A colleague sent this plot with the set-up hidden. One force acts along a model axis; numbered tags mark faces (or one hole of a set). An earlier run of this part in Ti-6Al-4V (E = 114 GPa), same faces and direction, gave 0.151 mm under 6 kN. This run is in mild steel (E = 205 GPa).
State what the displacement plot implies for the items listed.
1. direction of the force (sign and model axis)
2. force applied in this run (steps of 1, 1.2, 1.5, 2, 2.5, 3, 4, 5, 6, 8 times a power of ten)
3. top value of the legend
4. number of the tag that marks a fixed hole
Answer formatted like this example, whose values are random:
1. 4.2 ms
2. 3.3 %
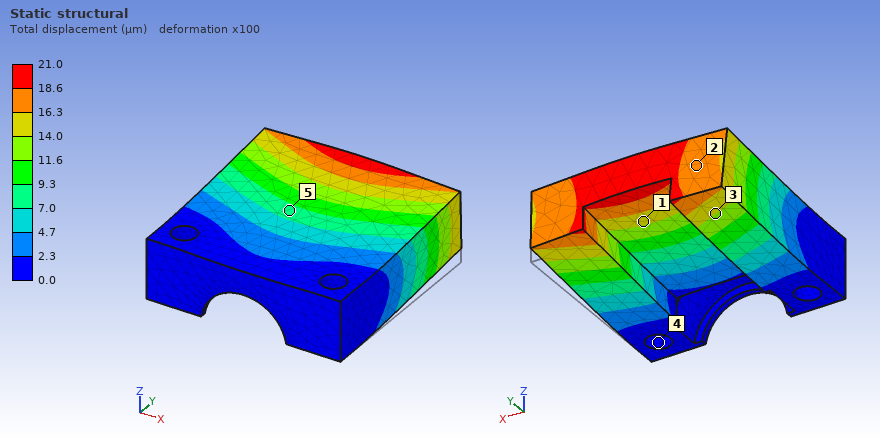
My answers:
1. +Z
2. 1.5 kN
3. 21.0 µm
4. 4
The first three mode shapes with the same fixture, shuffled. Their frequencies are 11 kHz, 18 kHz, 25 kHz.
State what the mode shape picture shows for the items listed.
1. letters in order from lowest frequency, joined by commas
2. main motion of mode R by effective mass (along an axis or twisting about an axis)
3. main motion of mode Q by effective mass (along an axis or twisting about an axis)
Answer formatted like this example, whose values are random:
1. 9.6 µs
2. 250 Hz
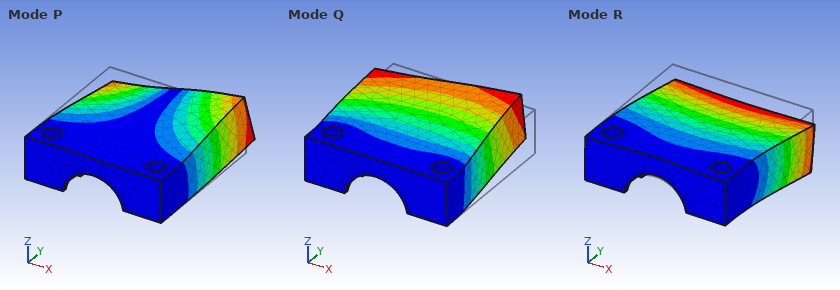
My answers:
1. R, P, Q
2. along Z
3. along X
